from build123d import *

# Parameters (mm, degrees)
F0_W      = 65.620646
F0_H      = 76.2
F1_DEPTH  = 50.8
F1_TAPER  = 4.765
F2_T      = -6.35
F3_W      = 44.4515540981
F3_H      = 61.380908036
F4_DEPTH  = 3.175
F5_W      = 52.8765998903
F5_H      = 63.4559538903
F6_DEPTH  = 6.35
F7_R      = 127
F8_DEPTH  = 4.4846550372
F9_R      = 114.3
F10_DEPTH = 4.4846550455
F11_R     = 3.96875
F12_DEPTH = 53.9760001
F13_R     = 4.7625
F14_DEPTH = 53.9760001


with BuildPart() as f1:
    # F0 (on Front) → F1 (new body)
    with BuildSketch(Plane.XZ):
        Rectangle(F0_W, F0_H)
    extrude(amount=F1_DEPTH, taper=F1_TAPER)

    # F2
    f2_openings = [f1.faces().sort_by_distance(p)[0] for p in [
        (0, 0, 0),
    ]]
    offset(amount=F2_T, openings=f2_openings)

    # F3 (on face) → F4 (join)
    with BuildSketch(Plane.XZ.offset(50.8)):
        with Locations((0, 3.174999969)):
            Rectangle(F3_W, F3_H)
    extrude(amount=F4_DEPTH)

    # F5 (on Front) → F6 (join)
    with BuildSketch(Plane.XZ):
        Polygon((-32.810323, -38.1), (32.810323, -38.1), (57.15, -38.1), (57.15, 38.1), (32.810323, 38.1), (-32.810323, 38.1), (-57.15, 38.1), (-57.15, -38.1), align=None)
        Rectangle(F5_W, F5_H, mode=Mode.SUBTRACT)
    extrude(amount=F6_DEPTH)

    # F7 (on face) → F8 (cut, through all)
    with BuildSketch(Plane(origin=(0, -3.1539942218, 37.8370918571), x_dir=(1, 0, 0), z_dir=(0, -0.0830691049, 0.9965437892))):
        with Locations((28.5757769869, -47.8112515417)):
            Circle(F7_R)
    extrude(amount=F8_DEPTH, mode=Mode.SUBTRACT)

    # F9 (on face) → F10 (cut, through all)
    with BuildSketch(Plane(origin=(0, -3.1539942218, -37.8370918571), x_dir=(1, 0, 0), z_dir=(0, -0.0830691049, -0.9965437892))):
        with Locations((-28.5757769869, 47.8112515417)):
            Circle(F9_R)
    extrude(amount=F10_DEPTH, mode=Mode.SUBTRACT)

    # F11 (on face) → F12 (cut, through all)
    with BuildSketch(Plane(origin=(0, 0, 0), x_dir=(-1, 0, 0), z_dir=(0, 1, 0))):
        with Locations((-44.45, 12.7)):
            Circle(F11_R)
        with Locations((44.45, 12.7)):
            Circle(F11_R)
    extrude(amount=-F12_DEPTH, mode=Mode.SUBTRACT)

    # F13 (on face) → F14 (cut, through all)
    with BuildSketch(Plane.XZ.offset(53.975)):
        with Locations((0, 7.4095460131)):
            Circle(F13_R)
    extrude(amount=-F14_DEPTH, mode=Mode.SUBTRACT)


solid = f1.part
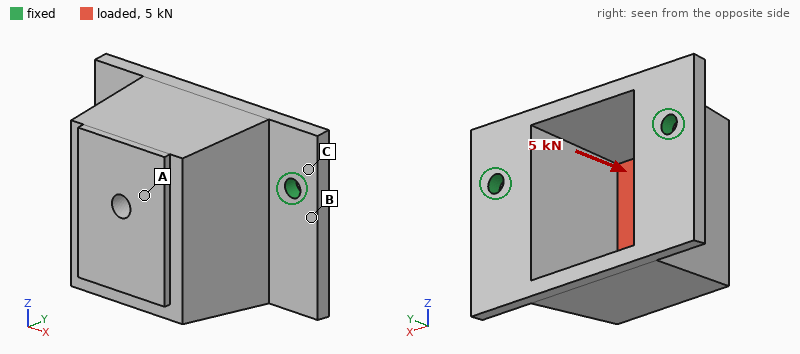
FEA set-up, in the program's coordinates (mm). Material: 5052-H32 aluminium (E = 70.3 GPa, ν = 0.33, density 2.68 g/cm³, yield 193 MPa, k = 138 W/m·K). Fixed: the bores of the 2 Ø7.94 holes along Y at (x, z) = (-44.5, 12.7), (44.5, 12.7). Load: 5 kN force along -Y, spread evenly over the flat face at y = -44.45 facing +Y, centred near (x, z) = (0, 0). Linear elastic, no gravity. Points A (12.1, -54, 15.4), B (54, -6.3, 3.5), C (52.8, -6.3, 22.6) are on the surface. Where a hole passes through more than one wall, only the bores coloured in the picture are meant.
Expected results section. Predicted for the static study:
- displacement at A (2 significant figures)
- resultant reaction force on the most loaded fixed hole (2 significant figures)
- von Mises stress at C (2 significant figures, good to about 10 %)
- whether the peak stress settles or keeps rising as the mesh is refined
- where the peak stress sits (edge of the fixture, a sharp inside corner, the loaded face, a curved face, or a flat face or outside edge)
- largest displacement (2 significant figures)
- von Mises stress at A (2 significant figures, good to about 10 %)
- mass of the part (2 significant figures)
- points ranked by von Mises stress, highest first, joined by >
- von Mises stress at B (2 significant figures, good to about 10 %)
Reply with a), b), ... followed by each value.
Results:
a) 0.17 mm
b) 2.7 kN
c) 26 MPa
d) keeps rising
e) edge of the fixture
f) 0.25 mm
g) 12 MPa
h) 330 g
i) B > C > A
j) 55 MPa
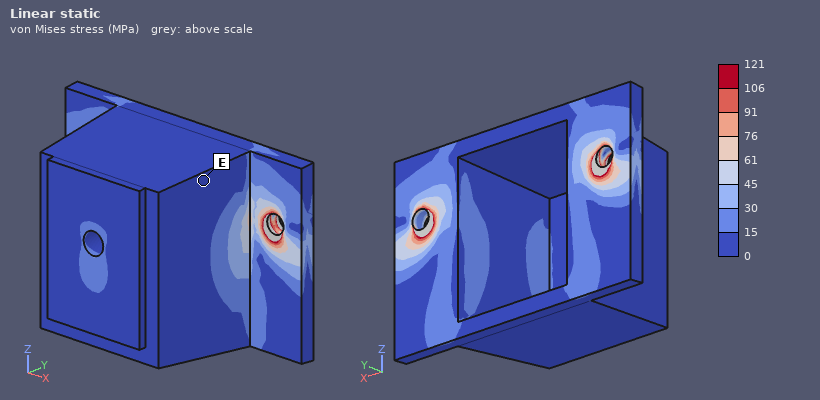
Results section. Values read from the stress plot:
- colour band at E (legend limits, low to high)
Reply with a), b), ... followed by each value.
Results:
a) 0 to 15 MPa
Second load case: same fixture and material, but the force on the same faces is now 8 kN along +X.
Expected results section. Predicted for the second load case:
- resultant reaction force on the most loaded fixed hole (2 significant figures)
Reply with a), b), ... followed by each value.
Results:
a) 6.0 kN
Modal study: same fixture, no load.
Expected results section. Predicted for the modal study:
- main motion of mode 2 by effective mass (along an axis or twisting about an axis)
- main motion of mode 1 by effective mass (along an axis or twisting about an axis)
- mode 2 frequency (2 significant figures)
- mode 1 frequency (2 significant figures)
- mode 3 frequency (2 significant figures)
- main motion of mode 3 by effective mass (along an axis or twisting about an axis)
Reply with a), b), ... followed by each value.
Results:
a) along X
b) along Z
c) 3300 Hz
d) 960 Hz
e) 3600 Hz
f) twisting about Z
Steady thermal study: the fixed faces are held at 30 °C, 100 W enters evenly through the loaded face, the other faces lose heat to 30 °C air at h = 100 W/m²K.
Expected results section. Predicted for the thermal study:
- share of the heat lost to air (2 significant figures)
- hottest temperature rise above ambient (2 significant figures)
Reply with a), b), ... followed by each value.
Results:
a) 59 %
b) 32 K
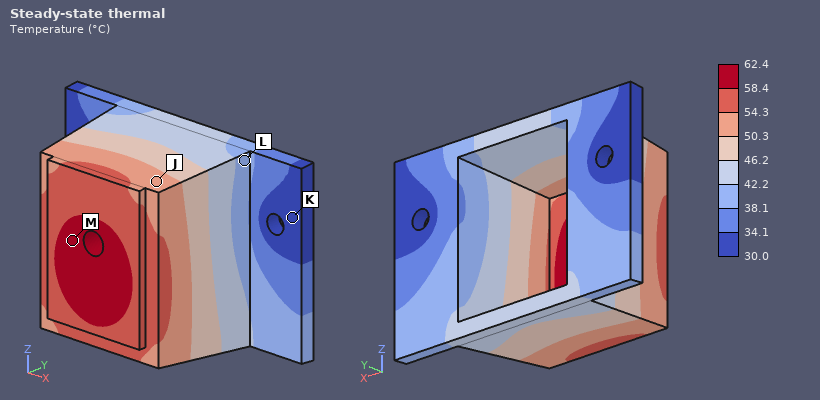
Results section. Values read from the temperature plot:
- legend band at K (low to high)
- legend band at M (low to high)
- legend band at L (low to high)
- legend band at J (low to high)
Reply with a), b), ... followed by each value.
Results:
a) 30.0 to 34.1 °C
b) 58.4 to 62.4 °C
c) 38.1 to 42.2 °C
d) 50.3 to 54.3 °C
